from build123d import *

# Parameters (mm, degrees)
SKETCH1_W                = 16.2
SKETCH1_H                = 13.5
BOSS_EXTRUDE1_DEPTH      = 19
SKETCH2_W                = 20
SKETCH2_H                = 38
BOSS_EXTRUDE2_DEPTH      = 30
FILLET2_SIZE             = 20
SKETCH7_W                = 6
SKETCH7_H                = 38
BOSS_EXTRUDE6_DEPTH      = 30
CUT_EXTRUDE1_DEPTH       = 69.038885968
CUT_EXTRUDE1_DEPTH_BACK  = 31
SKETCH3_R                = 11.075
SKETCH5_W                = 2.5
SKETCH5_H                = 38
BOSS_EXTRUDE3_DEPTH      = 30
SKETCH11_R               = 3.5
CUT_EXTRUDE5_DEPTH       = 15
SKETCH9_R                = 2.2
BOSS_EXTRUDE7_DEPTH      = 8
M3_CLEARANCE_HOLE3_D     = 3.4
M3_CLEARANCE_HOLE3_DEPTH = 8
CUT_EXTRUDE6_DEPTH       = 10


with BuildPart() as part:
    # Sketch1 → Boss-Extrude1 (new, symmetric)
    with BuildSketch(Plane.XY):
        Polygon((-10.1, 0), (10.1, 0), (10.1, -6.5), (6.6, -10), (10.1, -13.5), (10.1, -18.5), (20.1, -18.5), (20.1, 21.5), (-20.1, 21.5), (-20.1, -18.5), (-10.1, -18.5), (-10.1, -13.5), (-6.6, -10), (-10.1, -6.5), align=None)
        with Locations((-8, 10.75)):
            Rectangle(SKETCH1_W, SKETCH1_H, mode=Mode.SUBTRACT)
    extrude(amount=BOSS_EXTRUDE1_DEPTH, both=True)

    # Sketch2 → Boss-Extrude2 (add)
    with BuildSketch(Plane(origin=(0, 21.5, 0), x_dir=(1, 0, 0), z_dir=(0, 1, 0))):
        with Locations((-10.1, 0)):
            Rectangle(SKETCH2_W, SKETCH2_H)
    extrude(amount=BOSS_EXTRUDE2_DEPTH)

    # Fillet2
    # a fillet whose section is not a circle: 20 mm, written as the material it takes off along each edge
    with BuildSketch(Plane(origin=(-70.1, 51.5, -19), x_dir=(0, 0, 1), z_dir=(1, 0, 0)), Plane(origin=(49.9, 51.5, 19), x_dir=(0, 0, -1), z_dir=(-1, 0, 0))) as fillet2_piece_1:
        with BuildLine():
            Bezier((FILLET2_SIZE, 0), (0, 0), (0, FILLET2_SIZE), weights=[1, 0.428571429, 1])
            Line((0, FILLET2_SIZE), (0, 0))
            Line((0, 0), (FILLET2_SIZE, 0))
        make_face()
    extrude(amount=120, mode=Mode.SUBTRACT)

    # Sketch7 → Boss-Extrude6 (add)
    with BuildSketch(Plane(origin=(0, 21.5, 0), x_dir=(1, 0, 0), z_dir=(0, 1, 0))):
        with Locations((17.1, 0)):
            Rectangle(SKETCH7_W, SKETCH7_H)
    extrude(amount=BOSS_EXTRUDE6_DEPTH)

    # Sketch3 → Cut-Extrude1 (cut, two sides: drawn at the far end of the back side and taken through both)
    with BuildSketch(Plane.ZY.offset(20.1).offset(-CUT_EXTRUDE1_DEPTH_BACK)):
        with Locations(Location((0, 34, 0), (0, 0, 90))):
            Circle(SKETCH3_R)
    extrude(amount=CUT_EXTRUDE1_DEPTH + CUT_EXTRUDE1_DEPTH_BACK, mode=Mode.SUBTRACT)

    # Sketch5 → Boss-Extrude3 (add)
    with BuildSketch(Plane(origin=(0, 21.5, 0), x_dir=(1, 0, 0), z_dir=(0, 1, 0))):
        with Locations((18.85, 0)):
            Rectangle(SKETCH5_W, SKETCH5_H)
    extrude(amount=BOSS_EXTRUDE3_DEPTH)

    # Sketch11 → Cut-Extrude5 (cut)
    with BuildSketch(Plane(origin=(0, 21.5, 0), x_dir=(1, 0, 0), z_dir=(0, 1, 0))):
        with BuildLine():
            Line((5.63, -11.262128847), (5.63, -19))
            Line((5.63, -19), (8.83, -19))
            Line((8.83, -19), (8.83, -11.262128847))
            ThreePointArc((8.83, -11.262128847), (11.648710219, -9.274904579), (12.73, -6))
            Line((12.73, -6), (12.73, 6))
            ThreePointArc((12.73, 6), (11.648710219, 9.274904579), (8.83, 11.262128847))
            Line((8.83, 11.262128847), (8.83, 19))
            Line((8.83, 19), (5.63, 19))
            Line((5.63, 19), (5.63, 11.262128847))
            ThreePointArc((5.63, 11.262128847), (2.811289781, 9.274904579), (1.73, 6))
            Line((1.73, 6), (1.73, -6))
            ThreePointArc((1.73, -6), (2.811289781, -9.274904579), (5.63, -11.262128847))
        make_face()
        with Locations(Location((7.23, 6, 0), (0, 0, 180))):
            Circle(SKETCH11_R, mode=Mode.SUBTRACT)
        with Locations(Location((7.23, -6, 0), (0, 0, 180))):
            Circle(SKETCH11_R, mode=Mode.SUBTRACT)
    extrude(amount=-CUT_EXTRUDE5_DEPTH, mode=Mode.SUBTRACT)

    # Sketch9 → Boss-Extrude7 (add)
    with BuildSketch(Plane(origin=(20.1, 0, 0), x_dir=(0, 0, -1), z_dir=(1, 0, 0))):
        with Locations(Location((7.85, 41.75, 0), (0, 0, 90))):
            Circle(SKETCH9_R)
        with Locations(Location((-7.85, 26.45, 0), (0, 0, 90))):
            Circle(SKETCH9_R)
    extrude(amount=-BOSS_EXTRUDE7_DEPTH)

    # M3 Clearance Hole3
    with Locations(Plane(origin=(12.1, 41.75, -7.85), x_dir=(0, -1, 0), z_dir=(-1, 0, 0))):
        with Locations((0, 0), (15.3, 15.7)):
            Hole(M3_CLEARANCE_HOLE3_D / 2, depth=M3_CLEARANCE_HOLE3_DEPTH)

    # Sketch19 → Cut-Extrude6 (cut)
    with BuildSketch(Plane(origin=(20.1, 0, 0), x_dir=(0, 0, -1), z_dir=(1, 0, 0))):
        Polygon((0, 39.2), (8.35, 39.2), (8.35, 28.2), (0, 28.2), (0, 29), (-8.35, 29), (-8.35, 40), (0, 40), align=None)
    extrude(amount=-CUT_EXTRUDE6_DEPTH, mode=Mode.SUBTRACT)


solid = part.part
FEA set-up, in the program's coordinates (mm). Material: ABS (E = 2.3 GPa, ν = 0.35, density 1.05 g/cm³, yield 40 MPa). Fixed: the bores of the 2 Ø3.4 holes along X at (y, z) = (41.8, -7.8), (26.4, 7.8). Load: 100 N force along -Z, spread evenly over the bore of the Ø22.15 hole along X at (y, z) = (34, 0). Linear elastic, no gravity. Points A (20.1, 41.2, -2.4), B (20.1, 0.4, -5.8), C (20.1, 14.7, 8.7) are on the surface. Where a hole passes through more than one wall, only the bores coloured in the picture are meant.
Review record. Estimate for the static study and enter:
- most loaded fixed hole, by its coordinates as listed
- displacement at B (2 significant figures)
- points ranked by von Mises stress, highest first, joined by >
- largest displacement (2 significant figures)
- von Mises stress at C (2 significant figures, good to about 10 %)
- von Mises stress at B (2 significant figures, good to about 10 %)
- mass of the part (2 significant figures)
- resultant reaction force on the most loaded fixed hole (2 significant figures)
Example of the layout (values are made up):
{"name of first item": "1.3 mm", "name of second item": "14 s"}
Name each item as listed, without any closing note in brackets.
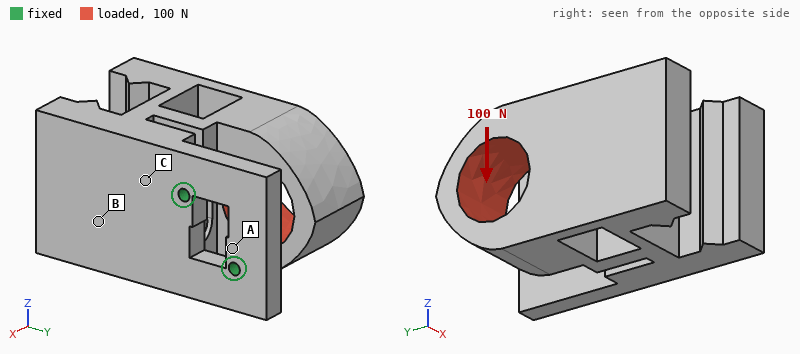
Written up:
{"most loaded fixed hole, by its coordinates as listed": "(26.4, 7.8)", "displacement at B": "0.32 mm", "points ranked by von Mises stress, highest first, joined by >": "C > B > A", "largest displacement": "1.0 mm", "von Mises stress at C": "5.4 MPa", "von Mises stress at B": "3.1 MPa", "mass of the part": "55 g", "resultant reaction force on the most loaded fixed hole": "110 N"}
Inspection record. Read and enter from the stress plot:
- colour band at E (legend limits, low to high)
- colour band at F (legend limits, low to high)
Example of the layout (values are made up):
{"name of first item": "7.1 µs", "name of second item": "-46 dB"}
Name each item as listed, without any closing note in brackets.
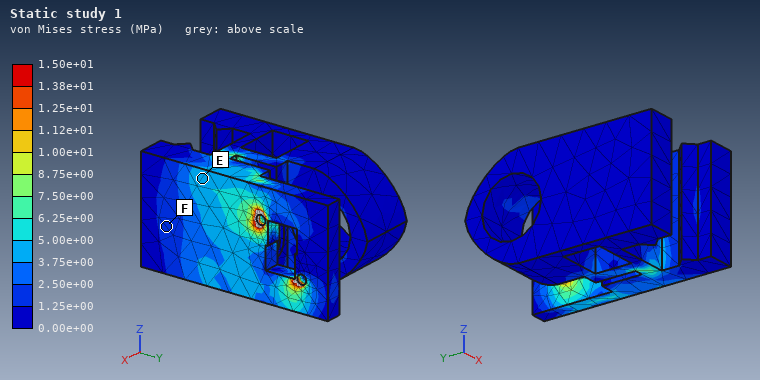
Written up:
{"colour band at E": "3.75e+00 to 5.00e+00 MPa", "colour band at F": "1.25e+00 to 2.50e+00 MPa"}
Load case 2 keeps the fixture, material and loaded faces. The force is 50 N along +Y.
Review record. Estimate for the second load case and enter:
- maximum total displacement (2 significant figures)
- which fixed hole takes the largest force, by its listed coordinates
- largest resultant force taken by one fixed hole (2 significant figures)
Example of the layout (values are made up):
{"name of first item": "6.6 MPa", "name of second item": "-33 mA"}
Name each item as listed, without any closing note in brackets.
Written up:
{"maximum total displacement": "0.98 mm", "which fixed hole takes the largest force, by its listed coordinates": "(26.4, 7.8)", "largest resultant force taken by one fixed hole": "36 N"}
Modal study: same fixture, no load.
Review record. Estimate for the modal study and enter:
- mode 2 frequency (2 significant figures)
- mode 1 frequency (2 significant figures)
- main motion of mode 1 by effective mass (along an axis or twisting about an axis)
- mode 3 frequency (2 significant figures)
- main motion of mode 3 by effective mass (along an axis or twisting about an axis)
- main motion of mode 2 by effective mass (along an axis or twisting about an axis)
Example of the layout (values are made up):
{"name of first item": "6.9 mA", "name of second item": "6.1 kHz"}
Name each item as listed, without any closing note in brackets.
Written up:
{"mode 2 frequency": "340 Hz", "mode 1 frequency": "210 Hz", "main motion of mode 1 by effective mass": "along Y", "mode 3 frequency": "540 Hz", "main motion of mode 3 by effective mass": "along X", "main motion of mode 2 by effective mass": "along Z"}
